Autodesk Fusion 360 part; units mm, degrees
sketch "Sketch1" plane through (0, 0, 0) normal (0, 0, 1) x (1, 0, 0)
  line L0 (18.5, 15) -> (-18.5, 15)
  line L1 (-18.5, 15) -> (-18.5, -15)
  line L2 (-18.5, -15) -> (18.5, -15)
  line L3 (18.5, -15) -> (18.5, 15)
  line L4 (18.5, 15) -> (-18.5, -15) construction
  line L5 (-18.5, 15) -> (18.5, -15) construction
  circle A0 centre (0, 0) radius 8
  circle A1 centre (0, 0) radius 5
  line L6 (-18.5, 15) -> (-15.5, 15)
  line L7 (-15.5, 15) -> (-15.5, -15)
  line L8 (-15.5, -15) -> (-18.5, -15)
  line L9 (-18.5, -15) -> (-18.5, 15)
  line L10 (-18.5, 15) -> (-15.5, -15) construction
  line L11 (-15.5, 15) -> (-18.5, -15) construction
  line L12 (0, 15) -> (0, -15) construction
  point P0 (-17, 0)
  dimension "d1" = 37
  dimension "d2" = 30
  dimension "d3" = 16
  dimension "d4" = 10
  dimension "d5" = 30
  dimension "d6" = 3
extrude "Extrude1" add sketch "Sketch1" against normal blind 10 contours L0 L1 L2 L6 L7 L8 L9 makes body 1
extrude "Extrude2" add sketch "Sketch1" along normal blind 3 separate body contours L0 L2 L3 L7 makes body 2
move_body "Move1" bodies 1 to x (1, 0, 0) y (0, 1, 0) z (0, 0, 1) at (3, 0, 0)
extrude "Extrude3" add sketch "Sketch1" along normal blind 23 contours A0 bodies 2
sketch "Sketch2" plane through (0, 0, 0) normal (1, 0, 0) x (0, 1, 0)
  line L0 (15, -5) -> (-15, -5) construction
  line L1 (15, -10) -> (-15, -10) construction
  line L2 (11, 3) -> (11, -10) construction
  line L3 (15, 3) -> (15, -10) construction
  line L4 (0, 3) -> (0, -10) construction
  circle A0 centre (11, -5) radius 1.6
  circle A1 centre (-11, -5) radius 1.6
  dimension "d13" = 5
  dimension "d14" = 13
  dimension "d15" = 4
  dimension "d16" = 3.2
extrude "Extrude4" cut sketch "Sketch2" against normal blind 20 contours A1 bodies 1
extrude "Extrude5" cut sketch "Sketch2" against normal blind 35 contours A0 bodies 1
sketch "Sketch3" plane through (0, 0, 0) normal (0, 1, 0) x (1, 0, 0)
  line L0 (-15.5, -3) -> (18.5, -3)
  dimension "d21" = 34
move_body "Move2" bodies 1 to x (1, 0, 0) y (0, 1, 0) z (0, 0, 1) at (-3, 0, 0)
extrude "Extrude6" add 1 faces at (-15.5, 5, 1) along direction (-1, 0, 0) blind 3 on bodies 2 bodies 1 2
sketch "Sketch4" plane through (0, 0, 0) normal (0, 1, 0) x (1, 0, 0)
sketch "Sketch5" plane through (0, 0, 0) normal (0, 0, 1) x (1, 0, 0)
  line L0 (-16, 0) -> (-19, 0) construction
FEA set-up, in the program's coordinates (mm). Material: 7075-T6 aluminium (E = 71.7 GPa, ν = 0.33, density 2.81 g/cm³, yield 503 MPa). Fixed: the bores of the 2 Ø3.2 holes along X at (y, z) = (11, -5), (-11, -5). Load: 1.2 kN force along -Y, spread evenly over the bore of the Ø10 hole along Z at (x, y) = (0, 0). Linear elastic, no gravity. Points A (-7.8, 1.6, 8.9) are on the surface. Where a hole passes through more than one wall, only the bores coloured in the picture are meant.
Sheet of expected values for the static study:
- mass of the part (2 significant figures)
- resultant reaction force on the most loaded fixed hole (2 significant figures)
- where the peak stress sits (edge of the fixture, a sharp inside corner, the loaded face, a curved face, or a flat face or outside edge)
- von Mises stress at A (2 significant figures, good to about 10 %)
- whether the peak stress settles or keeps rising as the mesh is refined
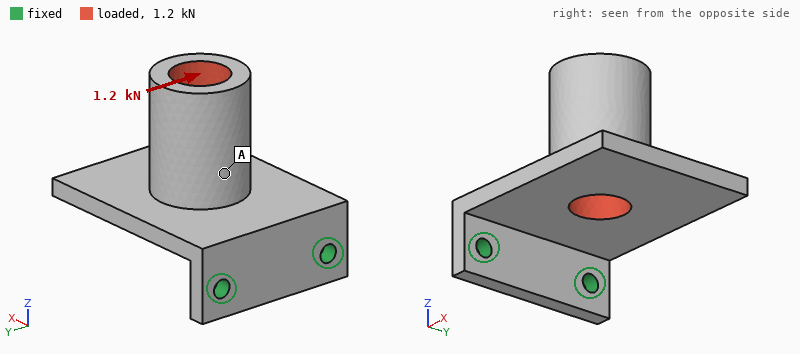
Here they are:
18 g
1.4 kN
edge of the fixture
21 MPa
keeps rising
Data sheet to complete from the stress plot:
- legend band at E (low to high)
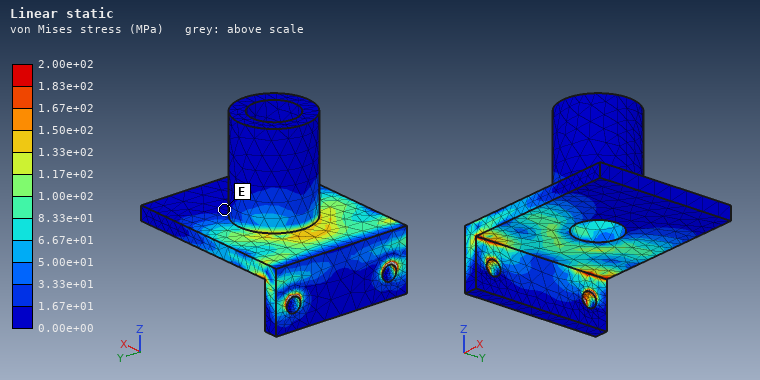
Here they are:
0.00e+00 to 1.67e+01 MPa
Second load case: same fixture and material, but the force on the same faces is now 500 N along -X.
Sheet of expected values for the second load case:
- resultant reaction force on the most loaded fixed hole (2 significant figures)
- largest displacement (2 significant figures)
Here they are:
250 N
0.66 mm
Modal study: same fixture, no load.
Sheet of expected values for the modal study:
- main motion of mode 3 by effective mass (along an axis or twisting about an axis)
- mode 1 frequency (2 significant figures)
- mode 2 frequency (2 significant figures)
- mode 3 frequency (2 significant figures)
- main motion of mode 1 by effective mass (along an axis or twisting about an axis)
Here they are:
along Y
1100 Hz
3900 Hz
5400 Hz
along Z
